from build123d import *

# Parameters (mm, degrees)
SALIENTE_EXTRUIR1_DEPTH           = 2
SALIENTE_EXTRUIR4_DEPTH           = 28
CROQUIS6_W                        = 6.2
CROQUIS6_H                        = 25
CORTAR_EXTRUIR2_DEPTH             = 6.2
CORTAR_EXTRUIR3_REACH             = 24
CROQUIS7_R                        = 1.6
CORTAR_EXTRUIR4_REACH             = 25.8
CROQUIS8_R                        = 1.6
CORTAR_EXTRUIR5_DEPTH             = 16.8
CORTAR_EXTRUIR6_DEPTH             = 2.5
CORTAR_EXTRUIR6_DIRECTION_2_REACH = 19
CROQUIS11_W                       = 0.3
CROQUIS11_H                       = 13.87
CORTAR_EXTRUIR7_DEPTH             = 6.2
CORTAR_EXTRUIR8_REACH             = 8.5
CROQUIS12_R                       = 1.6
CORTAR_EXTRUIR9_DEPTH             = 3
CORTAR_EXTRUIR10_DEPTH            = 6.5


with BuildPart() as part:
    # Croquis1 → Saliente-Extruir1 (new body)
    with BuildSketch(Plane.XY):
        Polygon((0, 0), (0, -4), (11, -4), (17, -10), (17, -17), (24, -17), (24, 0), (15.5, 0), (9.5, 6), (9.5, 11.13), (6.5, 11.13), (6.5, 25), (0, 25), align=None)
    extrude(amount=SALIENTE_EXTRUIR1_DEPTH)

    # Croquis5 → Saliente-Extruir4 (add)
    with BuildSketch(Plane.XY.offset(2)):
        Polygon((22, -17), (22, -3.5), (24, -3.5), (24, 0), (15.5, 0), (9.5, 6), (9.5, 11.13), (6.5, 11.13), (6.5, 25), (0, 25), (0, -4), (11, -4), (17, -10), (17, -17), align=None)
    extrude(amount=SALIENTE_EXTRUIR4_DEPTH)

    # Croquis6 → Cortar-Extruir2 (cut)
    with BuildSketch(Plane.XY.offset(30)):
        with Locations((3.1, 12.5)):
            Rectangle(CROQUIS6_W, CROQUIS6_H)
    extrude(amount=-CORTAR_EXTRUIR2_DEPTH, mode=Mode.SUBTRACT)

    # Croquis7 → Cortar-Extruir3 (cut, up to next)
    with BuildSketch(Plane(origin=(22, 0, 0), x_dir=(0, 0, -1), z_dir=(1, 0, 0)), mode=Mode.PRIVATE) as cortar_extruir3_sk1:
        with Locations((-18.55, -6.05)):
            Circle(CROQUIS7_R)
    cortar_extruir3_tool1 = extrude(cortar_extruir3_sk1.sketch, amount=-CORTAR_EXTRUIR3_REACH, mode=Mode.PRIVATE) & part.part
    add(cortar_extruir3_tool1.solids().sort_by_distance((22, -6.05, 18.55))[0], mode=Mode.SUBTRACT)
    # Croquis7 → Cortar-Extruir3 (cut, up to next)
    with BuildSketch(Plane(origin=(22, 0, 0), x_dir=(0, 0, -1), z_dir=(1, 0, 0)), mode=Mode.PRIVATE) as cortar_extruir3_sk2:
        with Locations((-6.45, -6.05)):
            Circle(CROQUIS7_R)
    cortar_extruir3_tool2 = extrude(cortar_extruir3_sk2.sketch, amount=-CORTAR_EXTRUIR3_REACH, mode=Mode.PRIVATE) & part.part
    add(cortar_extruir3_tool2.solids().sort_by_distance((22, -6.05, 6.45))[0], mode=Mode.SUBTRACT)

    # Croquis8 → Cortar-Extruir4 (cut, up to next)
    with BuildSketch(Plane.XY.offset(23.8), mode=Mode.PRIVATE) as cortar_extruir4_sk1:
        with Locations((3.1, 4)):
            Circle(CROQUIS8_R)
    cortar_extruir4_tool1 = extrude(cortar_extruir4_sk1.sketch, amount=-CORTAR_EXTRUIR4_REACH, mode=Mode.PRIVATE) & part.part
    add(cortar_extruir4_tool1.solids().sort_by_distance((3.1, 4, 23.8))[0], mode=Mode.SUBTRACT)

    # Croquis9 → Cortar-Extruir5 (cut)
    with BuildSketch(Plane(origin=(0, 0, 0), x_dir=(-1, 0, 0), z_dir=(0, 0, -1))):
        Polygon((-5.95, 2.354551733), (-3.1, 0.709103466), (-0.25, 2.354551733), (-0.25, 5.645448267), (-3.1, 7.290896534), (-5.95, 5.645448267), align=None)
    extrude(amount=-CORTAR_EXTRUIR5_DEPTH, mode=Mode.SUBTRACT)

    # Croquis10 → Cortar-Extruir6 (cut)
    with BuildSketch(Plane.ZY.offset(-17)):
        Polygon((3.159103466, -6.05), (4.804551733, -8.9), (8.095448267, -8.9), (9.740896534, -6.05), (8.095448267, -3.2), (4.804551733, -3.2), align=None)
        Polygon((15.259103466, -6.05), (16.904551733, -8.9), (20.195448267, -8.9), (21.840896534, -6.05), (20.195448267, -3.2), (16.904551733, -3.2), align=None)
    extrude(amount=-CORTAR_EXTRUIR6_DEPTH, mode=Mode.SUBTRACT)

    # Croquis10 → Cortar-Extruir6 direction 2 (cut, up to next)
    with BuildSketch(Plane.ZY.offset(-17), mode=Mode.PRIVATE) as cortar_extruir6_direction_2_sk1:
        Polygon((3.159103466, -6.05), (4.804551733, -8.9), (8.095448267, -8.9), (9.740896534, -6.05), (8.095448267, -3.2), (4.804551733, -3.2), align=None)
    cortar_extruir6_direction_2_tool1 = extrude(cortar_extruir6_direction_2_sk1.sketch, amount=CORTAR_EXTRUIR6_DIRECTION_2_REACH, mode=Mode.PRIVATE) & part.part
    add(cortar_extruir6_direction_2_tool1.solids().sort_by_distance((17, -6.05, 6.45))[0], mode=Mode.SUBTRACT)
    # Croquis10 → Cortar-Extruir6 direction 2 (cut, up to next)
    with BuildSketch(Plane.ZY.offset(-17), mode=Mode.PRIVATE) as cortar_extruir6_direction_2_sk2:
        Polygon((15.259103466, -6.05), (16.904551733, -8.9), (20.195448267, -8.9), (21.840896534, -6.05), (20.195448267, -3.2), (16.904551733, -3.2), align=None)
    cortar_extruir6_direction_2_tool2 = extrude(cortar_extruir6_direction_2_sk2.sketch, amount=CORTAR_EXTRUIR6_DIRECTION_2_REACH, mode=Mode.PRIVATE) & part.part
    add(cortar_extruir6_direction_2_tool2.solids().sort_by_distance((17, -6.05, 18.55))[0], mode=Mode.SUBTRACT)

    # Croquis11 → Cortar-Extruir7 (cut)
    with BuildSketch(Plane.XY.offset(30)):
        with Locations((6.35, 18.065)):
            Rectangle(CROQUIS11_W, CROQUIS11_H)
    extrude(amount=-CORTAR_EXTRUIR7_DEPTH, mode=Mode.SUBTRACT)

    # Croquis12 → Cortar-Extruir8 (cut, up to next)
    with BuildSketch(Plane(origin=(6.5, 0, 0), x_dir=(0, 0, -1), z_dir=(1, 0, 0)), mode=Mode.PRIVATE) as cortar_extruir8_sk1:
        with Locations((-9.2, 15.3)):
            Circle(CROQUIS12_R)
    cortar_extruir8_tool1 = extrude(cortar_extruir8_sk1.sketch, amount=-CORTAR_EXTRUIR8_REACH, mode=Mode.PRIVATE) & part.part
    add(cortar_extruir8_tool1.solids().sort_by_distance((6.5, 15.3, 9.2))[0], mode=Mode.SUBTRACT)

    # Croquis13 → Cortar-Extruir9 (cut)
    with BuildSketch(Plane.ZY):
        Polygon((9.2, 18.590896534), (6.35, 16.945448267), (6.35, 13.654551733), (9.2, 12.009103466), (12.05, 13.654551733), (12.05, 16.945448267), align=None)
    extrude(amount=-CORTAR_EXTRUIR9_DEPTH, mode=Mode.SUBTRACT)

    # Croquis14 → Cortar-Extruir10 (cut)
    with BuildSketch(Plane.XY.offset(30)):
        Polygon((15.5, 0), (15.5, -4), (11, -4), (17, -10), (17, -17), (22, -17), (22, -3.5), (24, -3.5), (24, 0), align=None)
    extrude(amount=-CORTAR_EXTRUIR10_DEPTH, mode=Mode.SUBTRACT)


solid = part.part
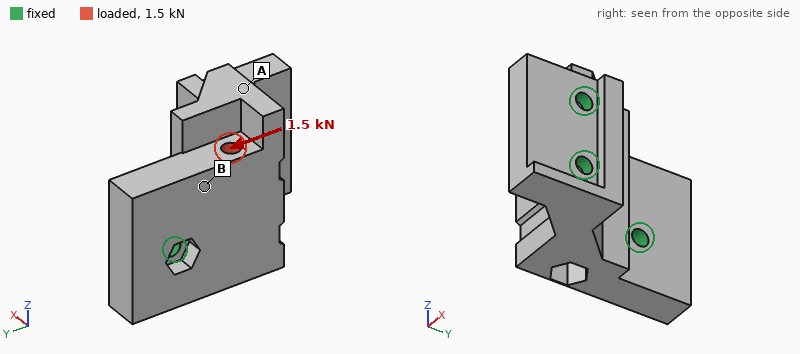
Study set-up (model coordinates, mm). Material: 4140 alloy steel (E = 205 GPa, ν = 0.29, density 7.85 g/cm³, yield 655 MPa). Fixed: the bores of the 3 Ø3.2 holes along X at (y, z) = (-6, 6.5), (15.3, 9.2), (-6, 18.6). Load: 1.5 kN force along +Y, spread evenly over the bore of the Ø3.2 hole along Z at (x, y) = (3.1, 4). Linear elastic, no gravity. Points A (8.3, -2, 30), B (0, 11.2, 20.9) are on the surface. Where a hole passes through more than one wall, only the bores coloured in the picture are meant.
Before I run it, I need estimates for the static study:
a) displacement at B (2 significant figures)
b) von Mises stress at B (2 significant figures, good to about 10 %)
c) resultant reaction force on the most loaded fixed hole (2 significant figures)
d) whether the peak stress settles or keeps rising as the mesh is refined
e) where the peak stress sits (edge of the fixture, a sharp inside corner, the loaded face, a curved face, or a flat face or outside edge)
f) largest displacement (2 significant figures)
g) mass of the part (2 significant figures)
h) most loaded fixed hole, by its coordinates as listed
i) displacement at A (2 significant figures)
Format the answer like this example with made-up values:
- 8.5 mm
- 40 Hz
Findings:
- 7.2 µm
- 21 MPa
- 1.4 kN
- keeps rising
- edge of the fixture
- 12 µm
- 70 g
- (15.3, 9.2)
- 8.8 µm
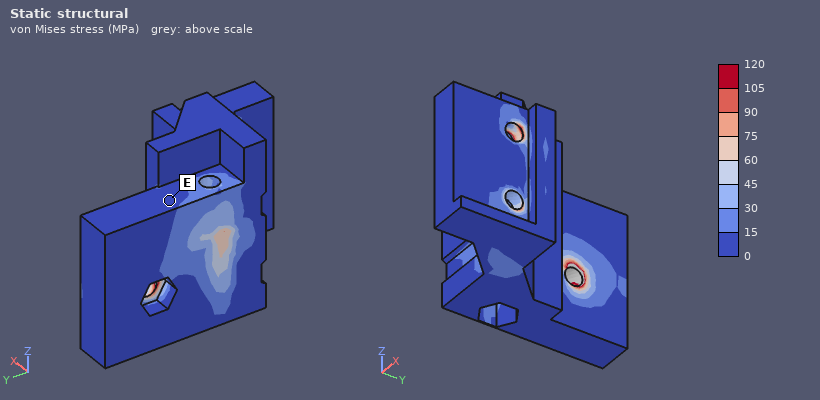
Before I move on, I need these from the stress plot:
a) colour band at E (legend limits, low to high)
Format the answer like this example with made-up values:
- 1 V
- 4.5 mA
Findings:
- 0 to 15 MPa
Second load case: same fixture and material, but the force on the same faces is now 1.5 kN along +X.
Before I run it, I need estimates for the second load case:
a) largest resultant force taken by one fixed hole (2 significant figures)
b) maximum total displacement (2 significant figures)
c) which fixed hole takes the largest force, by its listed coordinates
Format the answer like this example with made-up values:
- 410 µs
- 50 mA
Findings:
- 1.2 kN
- 11 µm
- (-6, 18.6)
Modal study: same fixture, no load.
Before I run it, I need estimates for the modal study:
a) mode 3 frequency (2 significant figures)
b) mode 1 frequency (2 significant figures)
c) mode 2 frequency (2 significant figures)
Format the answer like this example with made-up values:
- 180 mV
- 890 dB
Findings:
- 23 kHz
- 10 kHz
- 20 kHz
